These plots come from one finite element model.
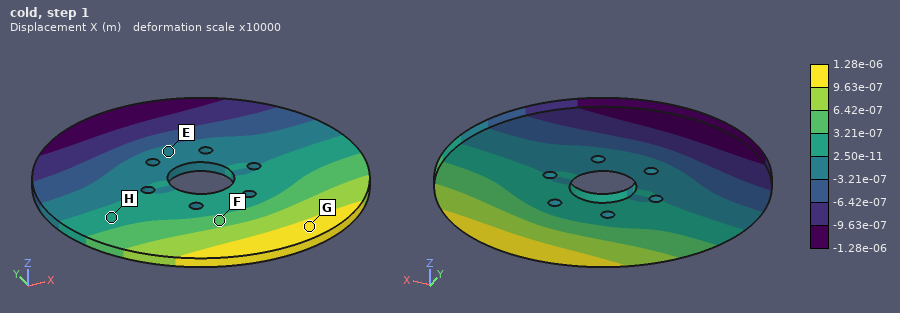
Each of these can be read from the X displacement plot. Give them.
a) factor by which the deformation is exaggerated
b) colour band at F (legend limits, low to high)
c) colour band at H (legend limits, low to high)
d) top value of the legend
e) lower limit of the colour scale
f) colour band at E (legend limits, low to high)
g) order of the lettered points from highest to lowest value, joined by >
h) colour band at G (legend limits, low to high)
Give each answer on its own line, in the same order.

10000
3.21e-07 to 6.42e-07 m
2.50e-11 to 3.21e-07 m
1.28e-06 m
-1.28e-06 m
-3.21e-07 to 2.50e-11 m
G > F > H > E
9.63e-07 to 1.28e-06 m
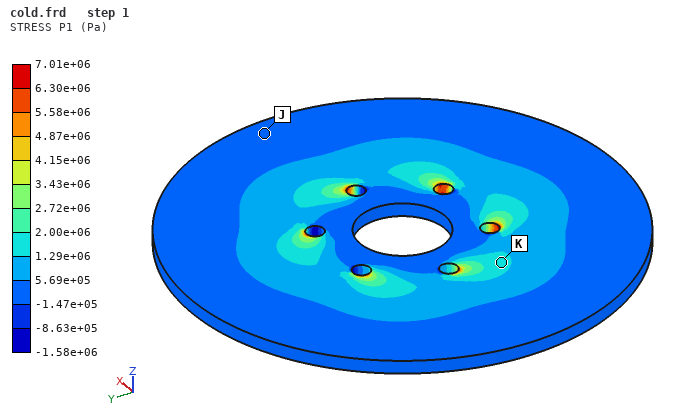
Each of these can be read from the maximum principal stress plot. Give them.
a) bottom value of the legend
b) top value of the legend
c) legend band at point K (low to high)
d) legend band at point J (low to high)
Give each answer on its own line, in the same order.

-1.58e+06 Pa
7.01e+06 Pa
1.29e+06 to 2.00e+06 Pa
-1.47e+05 to 5.69e+05 Pa
